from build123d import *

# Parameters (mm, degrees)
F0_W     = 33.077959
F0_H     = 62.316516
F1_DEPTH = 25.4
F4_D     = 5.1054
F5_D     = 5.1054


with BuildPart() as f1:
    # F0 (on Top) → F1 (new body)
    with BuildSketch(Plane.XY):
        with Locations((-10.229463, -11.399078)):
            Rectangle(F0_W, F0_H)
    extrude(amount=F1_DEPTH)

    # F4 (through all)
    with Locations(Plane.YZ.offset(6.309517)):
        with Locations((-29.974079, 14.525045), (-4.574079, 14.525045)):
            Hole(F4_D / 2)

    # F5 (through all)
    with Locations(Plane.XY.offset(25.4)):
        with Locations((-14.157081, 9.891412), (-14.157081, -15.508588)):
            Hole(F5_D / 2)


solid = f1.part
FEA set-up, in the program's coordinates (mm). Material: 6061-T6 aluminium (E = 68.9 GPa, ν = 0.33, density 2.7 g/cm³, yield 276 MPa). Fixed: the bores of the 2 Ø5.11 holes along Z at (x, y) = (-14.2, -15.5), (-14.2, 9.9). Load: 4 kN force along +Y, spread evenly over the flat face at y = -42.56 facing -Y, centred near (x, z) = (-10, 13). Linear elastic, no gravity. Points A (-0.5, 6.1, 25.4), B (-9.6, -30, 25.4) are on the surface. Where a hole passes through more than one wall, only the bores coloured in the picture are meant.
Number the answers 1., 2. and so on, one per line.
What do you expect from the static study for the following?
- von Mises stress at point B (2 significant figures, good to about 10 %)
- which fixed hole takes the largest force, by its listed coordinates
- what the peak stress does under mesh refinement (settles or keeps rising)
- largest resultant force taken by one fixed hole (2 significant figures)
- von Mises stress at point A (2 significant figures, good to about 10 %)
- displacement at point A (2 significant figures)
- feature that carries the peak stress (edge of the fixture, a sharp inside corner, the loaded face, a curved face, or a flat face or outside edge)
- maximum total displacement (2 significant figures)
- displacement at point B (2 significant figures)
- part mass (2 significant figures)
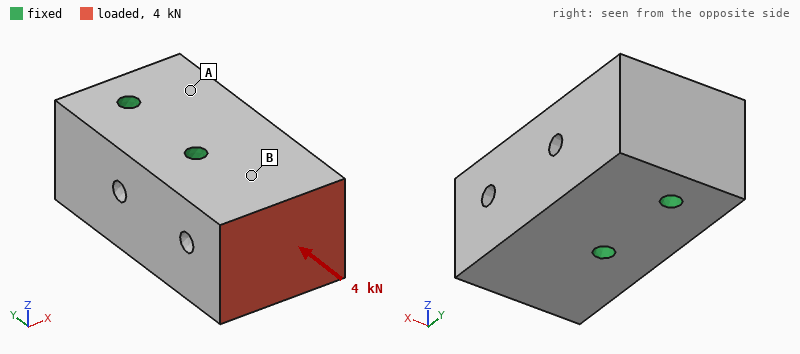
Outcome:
1. 5.3 MPa
2. (-14.2, -15.5)
3. keeps rising
4. 3.2 kN
5. 1.7 MPa
6. 0.76 µm
7. edge of the fixture
8. 4.3 µm
9. 2.0 µm
10. 130 g
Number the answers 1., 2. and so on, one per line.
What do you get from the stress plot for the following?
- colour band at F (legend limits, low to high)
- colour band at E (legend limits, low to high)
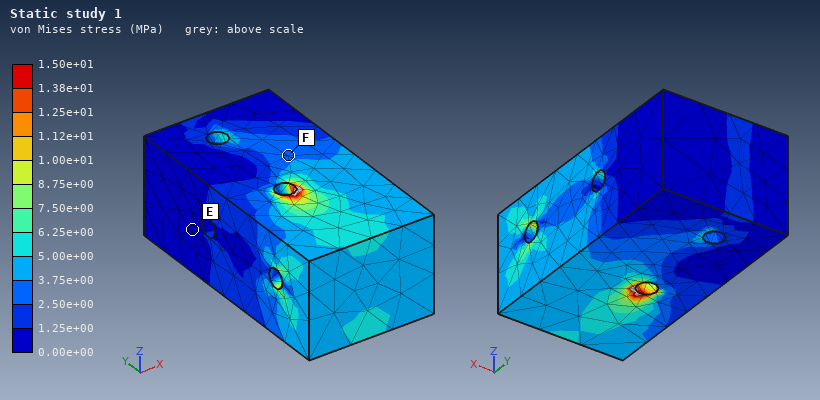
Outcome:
1. 2.50e+00 to 3.75e+00 MPa
2. 0.00e+00 to 1.25e+00 MPa
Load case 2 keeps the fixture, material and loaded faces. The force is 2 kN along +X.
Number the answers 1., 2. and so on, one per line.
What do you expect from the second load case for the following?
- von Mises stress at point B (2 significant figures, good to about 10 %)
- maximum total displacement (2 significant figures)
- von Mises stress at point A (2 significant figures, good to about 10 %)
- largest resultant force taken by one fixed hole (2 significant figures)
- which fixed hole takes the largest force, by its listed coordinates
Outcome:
1. 7.3 MPa
2. 13 µm
3. 3.9 MPa
4. 3.6 kN
5. (-14.2, -15.5)
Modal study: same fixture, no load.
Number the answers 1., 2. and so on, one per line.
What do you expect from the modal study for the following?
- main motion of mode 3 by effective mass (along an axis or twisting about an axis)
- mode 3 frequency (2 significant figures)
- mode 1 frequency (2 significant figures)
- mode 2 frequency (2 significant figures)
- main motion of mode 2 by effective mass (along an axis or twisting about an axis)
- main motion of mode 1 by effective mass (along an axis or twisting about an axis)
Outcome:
1. twisting about Y
2. 21 kHz
3. 14 kHz
4. 15 kHz
5. along Z
6. along X
